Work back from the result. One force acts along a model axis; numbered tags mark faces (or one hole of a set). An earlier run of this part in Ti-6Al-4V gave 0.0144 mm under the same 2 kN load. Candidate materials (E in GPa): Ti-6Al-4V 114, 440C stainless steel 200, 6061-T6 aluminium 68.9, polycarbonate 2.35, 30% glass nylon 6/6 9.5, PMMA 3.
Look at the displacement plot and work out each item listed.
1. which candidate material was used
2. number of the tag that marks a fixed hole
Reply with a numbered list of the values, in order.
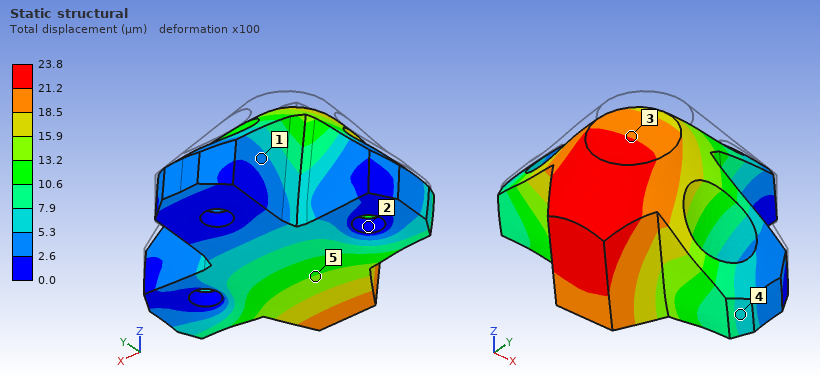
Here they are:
1. 6061-T6 aluminium
2. 2
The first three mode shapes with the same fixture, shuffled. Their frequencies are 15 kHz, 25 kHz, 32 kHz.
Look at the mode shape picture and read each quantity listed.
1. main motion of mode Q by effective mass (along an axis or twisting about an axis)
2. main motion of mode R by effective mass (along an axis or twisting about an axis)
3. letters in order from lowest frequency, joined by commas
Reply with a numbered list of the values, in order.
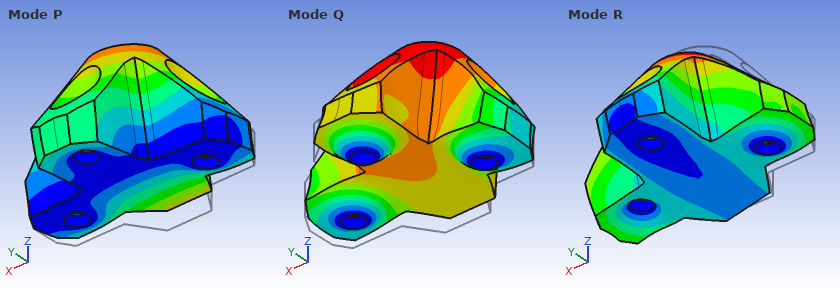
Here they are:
1. along Z
2. along X
3. P, R, Q
